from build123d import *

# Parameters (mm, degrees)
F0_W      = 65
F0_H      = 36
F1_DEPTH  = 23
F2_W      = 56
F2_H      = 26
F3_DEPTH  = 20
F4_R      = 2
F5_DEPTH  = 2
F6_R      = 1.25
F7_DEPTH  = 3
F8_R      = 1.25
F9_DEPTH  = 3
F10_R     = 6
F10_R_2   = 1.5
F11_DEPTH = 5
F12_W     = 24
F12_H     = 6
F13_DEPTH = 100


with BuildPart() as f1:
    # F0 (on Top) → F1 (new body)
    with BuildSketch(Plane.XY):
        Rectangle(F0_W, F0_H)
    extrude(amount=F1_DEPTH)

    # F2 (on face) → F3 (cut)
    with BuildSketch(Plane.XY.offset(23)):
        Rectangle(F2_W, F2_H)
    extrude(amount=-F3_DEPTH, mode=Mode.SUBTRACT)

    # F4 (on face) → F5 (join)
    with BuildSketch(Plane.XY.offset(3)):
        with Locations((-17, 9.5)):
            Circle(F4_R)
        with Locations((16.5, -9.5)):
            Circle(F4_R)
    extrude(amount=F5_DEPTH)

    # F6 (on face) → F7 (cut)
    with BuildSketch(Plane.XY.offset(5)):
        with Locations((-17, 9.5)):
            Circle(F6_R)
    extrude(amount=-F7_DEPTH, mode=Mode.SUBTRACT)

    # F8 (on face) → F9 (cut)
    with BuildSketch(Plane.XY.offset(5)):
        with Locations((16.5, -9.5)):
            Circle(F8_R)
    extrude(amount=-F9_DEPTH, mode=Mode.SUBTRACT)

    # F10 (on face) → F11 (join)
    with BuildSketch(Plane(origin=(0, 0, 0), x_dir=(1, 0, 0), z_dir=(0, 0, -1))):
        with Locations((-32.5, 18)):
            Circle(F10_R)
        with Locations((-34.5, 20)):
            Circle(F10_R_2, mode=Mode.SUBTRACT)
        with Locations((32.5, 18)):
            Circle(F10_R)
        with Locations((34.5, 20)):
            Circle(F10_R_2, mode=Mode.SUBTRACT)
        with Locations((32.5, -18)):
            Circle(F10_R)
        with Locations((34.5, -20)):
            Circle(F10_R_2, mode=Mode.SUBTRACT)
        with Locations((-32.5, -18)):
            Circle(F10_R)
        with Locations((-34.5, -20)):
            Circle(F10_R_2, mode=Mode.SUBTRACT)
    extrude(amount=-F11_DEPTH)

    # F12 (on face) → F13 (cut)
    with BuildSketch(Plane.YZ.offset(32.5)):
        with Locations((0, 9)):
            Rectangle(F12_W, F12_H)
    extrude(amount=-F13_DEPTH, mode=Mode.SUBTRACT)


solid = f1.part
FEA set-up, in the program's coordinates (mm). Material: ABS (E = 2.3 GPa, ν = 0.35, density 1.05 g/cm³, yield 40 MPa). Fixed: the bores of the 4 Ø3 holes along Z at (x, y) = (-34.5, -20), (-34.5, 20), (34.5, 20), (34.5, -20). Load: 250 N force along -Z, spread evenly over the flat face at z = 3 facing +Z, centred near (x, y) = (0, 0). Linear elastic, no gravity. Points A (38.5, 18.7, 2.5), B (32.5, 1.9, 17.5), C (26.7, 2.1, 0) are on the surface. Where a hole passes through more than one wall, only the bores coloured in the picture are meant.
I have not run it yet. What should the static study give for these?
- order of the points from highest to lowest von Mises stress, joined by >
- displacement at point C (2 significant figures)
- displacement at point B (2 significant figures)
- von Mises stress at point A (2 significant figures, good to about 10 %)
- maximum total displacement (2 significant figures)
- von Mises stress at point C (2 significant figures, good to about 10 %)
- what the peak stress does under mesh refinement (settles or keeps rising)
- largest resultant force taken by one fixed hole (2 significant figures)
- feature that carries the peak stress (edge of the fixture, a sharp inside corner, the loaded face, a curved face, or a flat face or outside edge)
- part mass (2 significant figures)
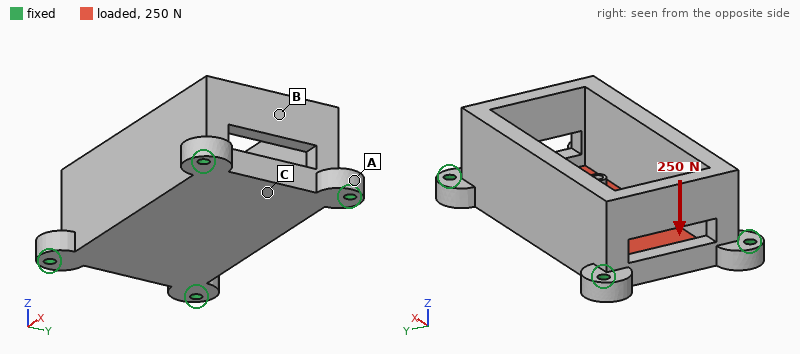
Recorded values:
C > A > B
0.067 mm
0.023 mm
1.5 MPa
0.15 mm
2.2 MPa
keeps rising
70 N
edge of the fixture
26 g
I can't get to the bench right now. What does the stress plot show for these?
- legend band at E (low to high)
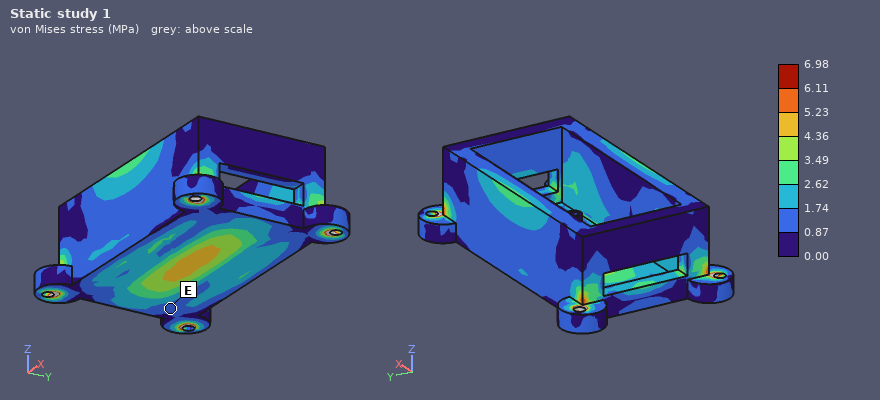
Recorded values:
0.87 to 1.74 MPa
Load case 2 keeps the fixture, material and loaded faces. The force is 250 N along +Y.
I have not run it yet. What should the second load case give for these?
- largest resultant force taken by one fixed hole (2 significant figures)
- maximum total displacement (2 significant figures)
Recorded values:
80 N
34 µm
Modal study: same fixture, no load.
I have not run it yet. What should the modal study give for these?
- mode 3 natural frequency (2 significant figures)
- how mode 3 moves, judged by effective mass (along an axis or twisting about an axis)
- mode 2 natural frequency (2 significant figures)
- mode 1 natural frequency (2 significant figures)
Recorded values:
2700 Hz
along Z
2200 Hz
2100 Hz
